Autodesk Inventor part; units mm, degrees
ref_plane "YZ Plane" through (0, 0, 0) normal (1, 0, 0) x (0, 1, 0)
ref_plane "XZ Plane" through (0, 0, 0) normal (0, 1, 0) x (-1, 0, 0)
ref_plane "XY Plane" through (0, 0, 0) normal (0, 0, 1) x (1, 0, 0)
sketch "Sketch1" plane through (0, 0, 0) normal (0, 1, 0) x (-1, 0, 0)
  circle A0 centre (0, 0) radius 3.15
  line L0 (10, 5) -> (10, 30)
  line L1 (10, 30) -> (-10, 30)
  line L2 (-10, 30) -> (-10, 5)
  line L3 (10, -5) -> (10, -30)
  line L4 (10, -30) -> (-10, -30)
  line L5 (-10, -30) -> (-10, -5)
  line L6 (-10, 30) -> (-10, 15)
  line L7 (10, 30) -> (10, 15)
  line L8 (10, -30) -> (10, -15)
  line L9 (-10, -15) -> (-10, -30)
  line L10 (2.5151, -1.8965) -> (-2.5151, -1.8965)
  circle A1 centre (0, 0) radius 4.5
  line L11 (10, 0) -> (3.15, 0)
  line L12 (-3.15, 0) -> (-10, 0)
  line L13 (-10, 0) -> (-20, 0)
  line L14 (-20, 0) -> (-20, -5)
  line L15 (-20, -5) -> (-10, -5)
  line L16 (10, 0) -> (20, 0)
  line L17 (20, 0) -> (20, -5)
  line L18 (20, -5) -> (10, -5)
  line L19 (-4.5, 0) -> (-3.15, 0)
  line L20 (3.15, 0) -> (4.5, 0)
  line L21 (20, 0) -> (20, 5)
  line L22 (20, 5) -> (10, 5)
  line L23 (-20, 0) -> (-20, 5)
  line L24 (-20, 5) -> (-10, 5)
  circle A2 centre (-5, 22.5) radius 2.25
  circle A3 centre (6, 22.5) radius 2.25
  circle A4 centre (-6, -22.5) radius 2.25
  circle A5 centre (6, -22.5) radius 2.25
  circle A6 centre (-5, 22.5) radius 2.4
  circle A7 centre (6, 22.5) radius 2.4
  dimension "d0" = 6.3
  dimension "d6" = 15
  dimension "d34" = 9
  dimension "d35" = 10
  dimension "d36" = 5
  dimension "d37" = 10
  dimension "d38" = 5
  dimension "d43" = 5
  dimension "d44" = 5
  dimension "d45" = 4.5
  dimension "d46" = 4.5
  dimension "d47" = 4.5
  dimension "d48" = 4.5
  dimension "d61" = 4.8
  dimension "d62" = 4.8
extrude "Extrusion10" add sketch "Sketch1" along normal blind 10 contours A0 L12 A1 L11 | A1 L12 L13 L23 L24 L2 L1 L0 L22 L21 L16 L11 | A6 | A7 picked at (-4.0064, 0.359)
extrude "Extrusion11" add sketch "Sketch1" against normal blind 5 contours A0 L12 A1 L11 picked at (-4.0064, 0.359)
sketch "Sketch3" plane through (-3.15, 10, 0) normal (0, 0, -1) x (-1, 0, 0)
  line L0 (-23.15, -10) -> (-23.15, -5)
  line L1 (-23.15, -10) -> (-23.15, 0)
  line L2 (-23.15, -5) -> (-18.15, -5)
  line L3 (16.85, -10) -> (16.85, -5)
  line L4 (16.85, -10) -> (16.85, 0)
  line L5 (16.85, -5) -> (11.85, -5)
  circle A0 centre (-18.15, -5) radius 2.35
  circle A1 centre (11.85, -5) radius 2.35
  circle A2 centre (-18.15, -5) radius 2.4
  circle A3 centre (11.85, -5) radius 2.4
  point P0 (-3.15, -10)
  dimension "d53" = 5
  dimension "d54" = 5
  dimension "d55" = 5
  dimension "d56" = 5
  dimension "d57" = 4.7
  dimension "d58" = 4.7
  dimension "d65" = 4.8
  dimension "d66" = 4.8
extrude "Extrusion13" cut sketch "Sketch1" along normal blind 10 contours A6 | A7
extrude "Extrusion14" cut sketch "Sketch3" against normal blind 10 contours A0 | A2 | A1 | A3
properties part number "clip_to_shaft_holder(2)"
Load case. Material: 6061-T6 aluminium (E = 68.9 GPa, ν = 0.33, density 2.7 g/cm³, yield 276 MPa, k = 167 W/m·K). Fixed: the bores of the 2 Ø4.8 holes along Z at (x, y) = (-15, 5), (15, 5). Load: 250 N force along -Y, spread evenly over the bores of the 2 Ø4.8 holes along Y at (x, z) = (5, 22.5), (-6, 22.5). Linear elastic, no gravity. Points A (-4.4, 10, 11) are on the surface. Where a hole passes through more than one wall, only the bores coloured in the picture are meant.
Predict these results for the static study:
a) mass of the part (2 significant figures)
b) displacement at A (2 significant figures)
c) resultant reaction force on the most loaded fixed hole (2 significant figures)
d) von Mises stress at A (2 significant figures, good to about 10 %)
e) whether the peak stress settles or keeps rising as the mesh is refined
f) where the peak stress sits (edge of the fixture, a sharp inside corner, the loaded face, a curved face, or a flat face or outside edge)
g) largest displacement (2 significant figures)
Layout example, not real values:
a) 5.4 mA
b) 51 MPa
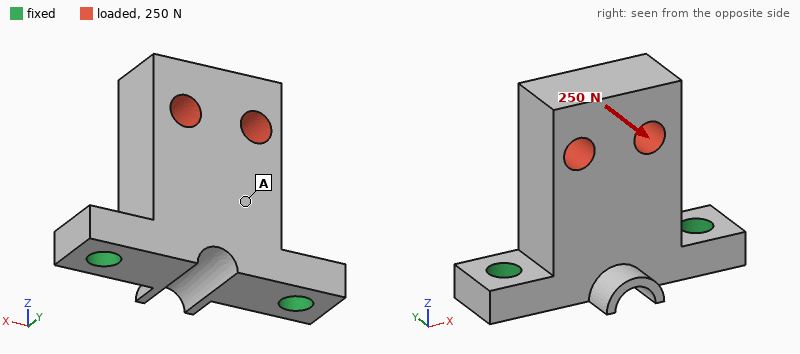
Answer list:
a) 17 g
b) 17 µm
c) 130 N
d) 8.0 MPa
e) keeps rising
f) edge of the fixture
g) 51 µm
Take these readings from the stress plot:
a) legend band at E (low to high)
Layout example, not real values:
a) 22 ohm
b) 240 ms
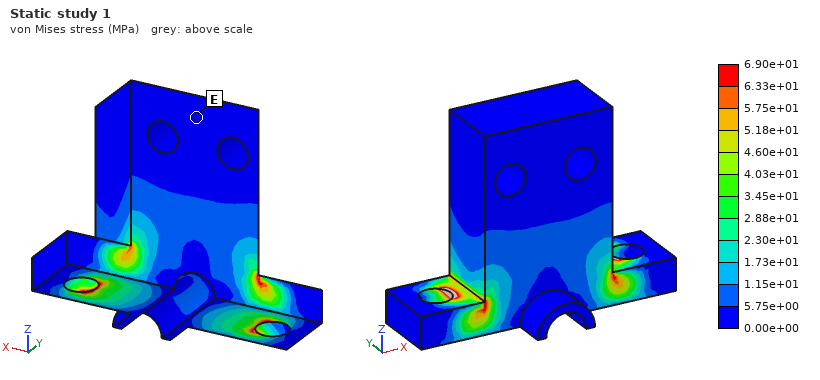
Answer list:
a) 0.00e+00 to 5.75e+00 MPa
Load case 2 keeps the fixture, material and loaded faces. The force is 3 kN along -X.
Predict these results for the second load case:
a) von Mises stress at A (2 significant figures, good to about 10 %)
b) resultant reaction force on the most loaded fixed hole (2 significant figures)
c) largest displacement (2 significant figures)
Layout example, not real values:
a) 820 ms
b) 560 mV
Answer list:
a) 39 MPa
b) 3.0 kN
c) 80 µm
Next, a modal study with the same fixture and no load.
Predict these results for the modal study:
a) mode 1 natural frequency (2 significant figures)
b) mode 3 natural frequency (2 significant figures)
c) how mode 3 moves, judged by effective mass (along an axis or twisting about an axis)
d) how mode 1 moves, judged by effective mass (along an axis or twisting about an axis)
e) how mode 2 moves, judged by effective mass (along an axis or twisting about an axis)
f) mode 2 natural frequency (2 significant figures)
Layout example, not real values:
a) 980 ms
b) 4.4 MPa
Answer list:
a) 4500 Hz
b) 20 kHz
c) along Z
d) along Y
e) along X
f) 12 kHz
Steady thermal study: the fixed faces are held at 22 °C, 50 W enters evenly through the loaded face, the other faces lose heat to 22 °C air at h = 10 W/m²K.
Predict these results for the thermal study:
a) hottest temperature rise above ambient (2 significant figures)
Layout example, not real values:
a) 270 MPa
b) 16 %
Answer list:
a) 51 K
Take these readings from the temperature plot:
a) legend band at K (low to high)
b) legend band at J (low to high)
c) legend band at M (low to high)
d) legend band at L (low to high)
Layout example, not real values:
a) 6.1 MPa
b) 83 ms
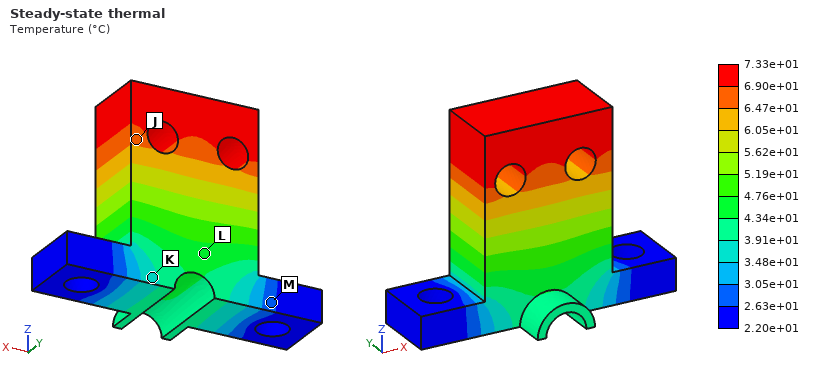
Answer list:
a) 3.48e+01 to 3.91e+01 °C
b) 6.47e+01 to 6.90e+01 °C
c) 2.63e+01 to 3.05e+01 °C
d) 4.34e+01 to 4.76e+01 °C
